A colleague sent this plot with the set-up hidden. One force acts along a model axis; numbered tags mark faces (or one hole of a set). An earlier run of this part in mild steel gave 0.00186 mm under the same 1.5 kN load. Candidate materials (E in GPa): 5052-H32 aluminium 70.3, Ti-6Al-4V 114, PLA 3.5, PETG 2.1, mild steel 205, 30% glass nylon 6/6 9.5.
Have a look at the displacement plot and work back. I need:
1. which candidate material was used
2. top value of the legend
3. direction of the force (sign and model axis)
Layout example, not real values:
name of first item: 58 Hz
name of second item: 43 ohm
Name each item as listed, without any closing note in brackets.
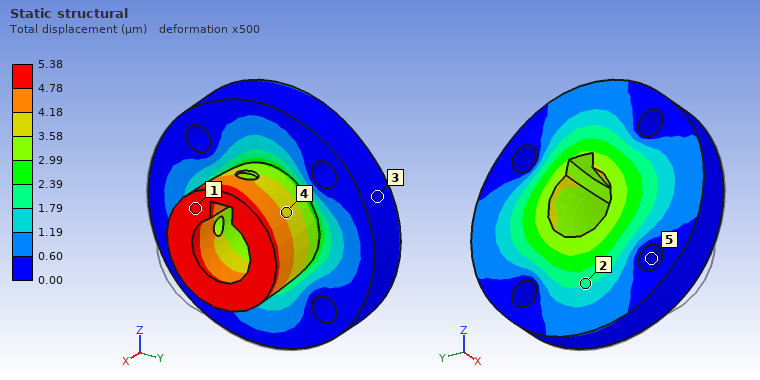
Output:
which candidate material was used: 5052-H32 aluminium
top value of the legend: 5.38 µm
direction of the force: -X
